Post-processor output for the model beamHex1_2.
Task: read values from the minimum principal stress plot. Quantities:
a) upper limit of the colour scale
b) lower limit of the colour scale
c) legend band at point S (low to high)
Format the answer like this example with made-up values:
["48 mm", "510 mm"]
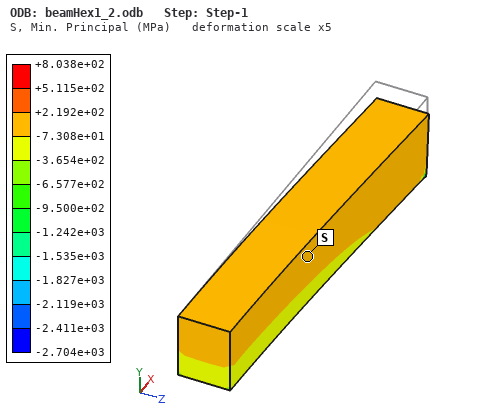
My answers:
["+8.038e+02 MPa", "-2.704e+03 MPa", "-7.308e+01 to +2.192e+02 MPa"]
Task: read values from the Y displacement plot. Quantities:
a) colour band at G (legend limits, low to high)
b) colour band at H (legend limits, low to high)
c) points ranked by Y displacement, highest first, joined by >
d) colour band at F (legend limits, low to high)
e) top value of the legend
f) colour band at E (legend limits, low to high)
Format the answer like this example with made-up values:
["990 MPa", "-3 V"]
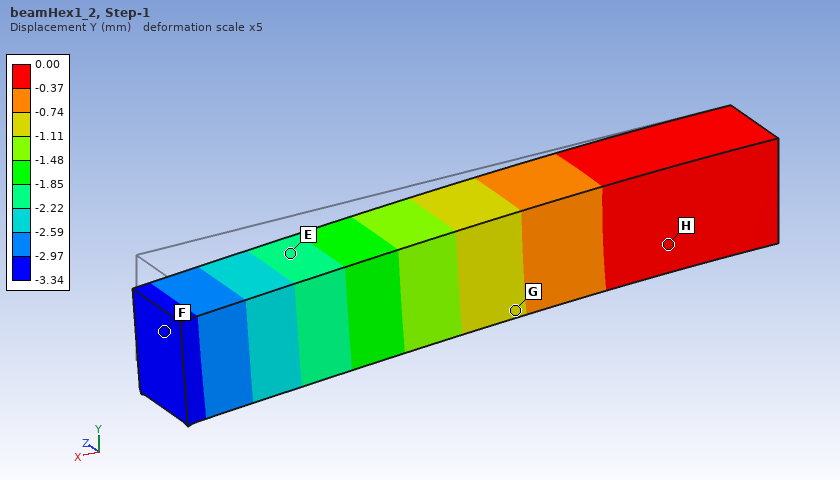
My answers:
["-1.11 to -0.74 mm", "-0.37 to 0.00 mm", "H > G > E > F", "-3.34 to -2.97 mm", "0.00 mm", "-2.22 to -1.85 mm"]
